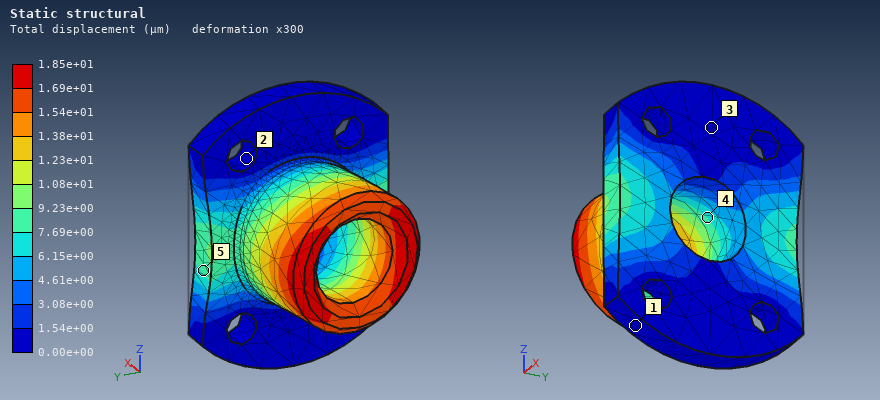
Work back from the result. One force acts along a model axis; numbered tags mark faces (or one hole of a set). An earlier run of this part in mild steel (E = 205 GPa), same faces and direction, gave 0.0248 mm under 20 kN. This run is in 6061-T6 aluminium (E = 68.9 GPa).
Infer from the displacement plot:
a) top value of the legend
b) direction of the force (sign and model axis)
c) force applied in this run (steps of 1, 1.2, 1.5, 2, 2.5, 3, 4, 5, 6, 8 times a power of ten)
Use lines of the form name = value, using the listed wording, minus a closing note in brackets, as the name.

top value of the legend = 1.85e+01 µm
direction of the force = -Y
force applied in this run = 5 kN
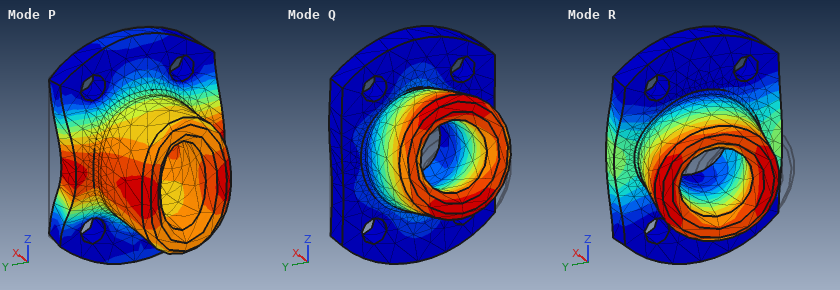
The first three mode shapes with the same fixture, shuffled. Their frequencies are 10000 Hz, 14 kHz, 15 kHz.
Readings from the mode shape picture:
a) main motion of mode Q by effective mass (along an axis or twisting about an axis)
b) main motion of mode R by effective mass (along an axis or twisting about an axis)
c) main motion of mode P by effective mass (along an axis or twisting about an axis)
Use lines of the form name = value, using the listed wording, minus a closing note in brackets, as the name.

main motion of mode Q by effective mass = along Z
main motion of mode R by effective mass = along Y
main motion of mode P by effective mass = along X
